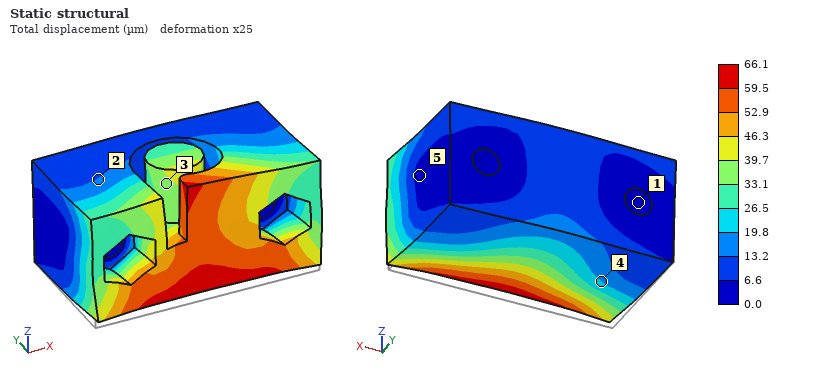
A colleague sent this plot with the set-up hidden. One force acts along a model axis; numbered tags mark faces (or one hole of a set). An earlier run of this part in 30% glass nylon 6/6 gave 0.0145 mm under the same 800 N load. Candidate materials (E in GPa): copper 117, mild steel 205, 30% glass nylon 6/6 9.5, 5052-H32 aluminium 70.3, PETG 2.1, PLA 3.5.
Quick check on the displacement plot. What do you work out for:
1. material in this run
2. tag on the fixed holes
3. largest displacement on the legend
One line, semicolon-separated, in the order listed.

PETG; 1; 66.1 µm
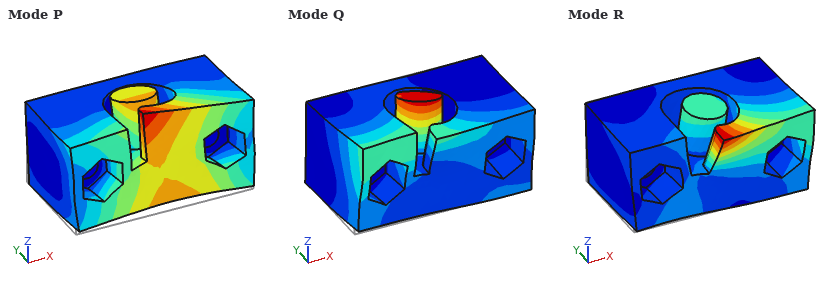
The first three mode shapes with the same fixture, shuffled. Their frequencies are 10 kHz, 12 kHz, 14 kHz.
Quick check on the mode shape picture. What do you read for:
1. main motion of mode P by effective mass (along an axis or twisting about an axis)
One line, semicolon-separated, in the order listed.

along Z
